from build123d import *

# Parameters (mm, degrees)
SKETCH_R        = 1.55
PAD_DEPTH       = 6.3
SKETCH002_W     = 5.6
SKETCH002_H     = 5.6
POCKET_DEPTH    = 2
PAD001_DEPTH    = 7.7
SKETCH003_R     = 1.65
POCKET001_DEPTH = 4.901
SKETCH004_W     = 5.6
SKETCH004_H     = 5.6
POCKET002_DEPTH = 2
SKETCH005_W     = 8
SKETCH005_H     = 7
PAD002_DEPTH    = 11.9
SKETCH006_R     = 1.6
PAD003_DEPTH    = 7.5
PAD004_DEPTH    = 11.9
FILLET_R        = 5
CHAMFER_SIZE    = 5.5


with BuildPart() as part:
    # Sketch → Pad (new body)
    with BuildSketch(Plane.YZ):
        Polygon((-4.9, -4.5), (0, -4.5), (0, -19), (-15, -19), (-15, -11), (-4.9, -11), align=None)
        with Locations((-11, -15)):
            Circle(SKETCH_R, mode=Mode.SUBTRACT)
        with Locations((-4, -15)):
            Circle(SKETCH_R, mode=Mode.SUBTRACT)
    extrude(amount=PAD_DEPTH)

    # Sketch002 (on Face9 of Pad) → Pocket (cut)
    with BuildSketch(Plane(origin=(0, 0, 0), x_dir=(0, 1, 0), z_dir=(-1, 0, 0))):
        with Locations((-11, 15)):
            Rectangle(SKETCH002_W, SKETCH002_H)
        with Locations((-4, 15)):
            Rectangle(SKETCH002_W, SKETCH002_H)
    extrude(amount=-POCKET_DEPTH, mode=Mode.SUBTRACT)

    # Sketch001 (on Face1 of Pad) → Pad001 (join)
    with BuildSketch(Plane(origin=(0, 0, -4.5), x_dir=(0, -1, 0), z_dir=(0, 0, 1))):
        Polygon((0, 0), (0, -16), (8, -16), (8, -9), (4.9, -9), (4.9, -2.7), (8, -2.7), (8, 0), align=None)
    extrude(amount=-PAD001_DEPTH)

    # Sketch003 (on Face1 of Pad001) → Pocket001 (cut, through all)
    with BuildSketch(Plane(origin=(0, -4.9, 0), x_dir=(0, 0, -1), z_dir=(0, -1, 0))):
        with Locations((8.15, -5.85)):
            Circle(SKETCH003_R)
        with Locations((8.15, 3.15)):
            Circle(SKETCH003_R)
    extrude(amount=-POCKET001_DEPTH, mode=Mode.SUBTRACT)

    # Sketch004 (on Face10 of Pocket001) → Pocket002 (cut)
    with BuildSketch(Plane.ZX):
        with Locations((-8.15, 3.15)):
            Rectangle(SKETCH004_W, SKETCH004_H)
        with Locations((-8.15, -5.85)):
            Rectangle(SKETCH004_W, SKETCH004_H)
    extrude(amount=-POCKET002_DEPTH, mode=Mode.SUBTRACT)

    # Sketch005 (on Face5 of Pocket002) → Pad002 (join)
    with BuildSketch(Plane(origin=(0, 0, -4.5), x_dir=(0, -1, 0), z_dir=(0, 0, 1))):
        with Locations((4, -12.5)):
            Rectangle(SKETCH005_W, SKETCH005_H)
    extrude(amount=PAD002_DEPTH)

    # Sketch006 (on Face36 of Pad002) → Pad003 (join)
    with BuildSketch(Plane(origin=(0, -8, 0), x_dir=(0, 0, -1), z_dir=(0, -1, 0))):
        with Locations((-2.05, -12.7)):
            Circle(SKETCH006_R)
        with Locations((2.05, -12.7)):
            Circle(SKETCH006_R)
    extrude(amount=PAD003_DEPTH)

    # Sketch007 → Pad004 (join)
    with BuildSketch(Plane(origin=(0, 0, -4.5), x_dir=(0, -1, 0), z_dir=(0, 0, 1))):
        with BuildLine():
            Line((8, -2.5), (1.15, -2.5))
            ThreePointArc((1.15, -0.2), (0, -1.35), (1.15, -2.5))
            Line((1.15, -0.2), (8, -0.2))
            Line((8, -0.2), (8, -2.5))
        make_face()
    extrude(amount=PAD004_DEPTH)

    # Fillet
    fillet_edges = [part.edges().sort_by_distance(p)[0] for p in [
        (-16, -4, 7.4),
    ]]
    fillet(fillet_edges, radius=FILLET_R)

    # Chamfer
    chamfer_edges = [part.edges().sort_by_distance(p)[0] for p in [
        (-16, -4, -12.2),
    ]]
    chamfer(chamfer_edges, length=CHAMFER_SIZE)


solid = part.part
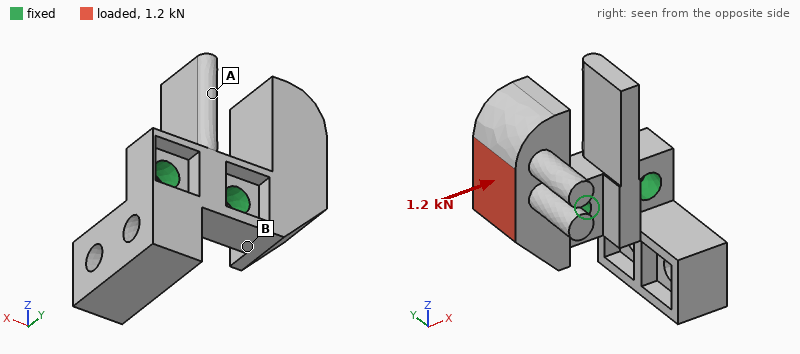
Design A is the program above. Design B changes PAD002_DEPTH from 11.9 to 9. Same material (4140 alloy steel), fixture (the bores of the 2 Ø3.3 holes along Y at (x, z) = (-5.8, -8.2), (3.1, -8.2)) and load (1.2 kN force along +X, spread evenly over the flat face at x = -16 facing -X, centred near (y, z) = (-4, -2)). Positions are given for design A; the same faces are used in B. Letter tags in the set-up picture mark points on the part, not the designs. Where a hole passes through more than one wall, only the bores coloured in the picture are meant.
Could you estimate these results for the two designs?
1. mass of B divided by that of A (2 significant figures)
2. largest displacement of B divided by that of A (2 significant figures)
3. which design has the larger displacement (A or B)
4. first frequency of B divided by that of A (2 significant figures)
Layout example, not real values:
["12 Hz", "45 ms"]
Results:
["0.93", "0.74", "A", "1.2"]
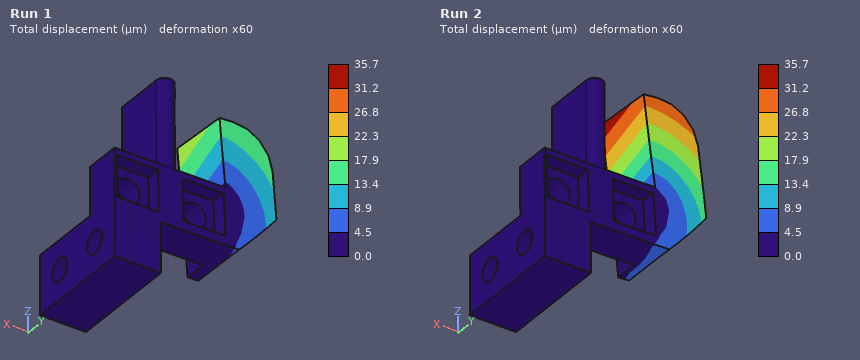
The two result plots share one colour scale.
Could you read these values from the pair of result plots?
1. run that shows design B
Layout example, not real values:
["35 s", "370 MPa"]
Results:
["Run 1"]
